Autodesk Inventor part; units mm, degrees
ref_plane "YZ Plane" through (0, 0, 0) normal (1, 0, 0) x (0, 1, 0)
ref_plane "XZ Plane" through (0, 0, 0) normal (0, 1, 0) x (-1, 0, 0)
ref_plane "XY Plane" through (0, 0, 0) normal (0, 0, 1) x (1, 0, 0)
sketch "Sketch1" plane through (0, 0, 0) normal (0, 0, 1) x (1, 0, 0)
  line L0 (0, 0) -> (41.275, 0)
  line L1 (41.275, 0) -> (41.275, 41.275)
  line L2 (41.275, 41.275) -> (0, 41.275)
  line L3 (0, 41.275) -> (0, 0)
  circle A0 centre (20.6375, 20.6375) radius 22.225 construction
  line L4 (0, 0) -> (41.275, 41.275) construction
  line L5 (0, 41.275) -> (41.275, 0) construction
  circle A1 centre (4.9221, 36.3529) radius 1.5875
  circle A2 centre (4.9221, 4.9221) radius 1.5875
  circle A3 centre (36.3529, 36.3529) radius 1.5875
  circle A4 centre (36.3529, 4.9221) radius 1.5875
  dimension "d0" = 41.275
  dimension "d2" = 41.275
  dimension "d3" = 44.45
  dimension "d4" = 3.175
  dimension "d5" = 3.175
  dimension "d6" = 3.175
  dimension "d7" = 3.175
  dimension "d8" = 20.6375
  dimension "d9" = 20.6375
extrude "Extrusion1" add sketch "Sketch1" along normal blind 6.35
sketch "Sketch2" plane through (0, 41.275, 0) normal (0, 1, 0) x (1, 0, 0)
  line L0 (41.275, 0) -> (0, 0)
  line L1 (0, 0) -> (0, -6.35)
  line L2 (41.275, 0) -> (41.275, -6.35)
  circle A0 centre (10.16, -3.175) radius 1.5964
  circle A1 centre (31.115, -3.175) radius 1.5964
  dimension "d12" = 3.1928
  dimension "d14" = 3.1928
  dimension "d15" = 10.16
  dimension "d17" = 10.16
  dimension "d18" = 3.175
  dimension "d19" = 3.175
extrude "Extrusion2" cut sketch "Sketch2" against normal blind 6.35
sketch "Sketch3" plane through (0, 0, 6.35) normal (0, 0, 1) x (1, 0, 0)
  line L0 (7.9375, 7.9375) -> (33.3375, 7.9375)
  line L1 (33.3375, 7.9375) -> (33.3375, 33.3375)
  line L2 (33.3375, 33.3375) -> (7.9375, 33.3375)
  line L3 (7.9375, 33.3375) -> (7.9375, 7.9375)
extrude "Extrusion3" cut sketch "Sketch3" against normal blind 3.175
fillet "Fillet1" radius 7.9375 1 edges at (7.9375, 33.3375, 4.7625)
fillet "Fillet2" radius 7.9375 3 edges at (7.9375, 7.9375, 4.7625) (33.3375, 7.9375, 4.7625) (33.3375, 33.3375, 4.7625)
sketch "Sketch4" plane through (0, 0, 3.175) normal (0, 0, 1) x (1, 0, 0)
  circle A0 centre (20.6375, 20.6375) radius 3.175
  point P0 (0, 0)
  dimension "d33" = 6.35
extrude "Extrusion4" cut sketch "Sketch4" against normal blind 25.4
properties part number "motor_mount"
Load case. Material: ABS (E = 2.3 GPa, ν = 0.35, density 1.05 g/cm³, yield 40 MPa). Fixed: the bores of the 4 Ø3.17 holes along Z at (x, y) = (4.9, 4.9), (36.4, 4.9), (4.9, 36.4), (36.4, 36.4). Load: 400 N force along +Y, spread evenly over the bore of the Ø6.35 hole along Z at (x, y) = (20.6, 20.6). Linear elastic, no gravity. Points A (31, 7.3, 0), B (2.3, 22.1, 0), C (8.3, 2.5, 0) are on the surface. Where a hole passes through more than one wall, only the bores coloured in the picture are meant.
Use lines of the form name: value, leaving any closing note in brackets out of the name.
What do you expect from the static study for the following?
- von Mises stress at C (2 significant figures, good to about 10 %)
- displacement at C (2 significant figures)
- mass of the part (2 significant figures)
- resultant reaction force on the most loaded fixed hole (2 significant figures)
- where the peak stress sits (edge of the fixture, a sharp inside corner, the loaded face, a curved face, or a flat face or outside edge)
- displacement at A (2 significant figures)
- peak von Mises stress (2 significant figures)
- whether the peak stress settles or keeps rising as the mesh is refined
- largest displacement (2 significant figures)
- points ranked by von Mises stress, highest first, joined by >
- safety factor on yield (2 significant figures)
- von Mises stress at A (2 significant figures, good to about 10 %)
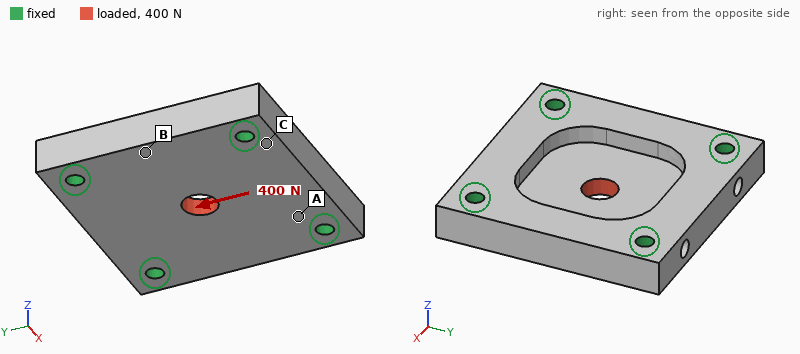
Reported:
von Mises stress at C: 1.9 MPa
displacement at C: 5.9 µm
mass of the part: 9.0 g
resultant reaction force on the most loaded fixed hole: 110 N
where the peak stress sits: the loaded face
displacement at A: 9.9 µm
peak von Mises stress: 11 MPa
whether the peak stress settles or keeps rising as the mesh is refined: settles
largest displacement: 37 µm
points ranked by von Mises stress, highest first, joined by >: A > C > B
safety factor on yield: 3.6
von Mises stress at A: 3.1 MPa
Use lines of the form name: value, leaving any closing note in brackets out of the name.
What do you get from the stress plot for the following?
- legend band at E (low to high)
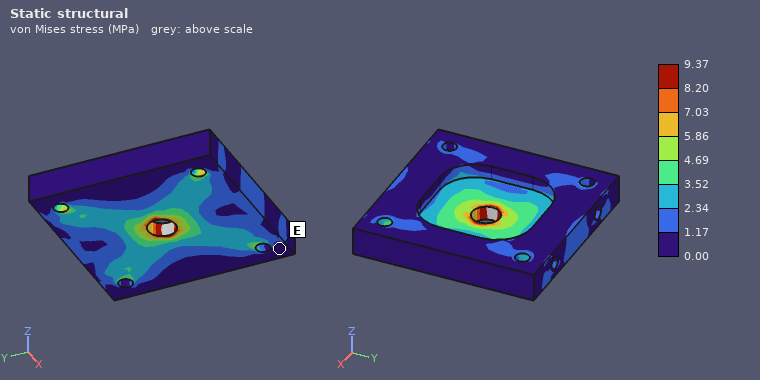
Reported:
legend band at E: 0.00 to 1.17 MPa
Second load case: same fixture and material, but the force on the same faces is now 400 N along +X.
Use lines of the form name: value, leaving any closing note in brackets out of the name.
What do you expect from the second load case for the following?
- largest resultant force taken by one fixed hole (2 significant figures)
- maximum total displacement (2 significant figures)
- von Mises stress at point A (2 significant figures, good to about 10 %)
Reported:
largest resultant force taken by one fixed hole: 110 N
maximum total displacement: 37 µm
von Mises stress at point A: 2.5 MPa
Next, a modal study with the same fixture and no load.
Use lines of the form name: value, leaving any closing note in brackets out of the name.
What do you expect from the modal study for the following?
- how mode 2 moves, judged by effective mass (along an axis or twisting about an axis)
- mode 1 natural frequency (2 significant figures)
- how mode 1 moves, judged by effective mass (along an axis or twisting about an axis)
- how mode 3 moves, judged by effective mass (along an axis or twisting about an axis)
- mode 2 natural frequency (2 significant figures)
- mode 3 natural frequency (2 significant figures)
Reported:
how mode 2 moves, judged by effective mass: twisting about X
mode 1 natural frequency: 5700 Hz
how mode 1 moves, judged by effective mass: along Z
how mode 3 moves, judged by effective mass: twisting about Y
mode 2 natural frequency: 7600 Hz
mode 3 natural frequency: 8100 Hz
